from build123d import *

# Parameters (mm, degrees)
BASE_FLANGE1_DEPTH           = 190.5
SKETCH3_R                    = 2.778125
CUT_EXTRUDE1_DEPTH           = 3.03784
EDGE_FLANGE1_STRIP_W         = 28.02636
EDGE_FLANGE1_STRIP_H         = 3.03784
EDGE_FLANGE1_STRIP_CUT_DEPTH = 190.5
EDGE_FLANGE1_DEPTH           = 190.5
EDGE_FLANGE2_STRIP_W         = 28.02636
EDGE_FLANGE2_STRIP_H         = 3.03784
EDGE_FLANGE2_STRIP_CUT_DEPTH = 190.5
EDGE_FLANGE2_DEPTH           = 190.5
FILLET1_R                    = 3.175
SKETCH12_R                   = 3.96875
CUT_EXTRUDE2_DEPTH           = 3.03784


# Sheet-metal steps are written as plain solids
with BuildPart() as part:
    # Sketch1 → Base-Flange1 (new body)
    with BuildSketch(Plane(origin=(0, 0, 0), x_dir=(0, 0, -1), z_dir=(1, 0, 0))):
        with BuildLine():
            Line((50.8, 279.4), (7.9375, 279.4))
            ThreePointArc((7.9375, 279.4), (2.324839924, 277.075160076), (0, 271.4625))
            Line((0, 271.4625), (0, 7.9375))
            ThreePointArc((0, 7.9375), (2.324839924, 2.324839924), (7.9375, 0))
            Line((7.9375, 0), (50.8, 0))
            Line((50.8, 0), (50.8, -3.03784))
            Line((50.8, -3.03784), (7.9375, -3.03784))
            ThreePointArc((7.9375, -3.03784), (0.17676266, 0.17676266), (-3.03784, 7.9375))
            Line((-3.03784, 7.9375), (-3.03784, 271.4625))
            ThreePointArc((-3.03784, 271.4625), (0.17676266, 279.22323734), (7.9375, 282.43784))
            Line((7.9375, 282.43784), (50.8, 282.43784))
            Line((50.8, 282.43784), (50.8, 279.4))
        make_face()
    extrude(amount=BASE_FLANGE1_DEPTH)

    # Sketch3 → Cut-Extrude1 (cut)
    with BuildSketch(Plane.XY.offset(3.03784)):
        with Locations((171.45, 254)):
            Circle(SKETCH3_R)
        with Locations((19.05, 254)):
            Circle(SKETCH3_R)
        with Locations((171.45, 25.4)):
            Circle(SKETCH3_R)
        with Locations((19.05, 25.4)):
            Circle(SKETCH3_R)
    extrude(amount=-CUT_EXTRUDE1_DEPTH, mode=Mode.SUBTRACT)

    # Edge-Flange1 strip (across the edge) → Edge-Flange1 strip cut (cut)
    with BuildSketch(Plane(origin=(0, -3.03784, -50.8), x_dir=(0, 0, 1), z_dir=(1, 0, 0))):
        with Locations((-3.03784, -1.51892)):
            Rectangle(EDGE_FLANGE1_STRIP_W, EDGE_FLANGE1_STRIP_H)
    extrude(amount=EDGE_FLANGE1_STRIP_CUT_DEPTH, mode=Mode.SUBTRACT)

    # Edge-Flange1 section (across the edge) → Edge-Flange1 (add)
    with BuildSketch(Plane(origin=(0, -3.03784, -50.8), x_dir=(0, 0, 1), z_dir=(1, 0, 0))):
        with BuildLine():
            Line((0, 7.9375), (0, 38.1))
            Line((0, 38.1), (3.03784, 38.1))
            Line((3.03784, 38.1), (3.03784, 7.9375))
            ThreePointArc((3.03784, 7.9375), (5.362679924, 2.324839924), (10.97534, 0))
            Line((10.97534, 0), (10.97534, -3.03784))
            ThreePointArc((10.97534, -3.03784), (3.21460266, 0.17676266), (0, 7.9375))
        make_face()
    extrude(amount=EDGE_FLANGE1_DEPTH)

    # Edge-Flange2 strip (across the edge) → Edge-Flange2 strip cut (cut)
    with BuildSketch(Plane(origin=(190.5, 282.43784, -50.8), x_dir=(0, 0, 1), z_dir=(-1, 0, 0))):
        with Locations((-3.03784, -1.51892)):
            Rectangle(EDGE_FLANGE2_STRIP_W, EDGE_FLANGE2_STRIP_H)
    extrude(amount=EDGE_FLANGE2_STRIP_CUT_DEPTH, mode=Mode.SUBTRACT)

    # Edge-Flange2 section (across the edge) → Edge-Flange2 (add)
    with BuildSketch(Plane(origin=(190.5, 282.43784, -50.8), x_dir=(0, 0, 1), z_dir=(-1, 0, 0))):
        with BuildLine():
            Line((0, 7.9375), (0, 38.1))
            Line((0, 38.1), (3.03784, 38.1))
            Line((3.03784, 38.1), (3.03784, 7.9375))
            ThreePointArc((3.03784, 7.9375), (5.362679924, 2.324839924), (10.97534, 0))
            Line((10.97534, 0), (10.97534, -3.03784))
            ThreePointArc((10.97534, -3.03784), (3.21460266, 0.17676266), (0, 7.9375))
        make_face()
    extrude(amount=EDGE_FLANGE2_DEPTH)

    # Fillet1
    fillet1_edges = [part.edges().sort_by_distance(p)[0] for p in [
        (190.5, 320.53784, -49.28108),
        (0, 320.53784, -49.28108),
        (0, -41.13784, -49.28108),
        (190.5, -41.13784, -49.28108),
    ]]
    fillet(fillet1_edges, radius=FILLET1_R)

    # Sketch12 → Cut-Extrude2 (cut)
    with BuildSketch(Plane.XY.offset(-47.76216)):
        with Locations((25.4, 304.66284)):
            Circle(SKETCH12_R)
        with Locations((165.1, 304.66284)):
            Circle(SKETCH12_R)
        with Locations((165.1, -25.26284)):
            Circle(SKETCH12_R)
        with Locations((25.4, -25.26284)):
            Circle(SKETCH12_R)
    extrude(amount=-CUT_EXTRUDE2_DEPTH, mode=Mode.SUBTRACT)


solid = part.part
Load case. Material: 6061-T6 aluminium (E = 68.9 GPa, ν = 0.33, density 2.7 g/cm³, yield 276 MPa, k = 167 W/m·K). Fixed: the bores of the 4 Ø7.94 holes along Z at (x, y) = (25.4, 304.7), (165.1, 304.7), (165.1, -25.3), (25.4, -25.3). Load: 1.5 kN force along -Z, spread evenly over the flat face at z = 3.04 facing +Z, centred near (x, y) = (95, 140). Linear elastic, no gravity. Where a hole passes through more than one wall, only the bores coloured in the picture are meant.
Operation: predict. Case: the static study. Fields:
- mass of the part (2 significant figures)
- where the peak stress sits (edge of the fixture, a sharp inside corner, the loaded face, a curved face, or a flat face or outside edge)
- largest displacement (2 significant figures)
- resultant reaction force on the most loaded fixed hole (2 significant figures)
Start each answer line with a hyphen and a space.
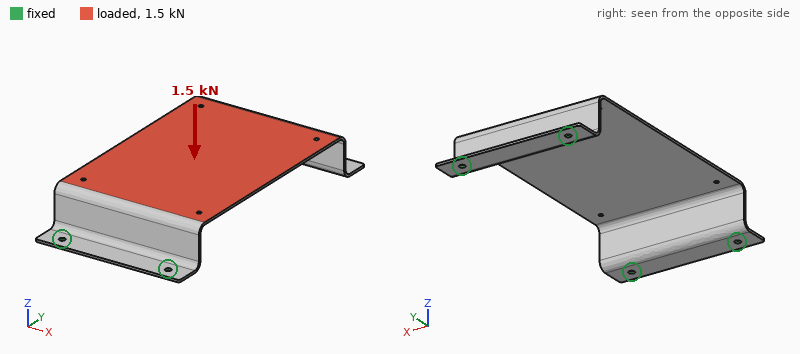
- 700 g
- a curved face
- 3.8 mm
- 640 N
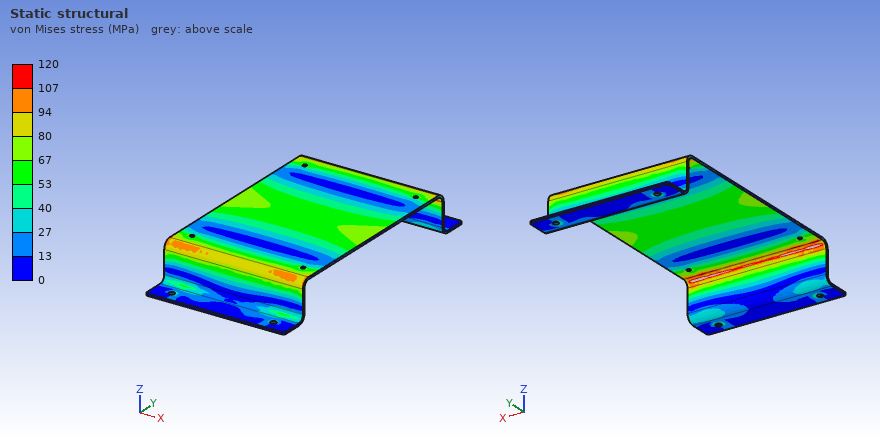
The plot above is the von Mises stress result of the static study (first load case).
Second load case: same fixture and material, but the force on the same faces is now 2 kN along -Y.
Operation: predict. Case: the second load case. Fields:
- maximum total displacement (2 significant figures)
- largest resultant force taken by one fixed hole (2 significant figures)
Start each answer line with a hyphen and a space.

- 2.0 mm
- 540 N
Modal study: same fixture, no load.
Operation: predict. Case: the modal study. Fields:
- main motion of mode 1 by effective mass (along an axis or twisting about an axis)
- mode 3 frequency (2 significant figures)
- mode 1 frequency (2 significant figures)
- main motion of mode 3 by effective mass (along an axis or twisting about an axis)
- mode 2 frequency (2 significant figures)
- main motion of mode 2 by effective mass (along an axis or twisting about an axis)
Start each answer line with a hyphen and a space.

- along Z
- 260 Hz
- 180 Hz
- twisting about Y
- 220 Hz
- along Y
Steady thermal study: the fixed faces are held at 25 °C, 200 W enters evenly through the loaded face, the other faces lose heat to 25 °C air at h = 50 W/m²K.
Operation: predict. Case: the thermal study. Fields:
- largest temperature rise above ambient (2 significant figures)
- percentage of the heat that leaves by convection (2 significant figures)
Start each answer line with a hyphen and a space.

- 53 K
- 82 %
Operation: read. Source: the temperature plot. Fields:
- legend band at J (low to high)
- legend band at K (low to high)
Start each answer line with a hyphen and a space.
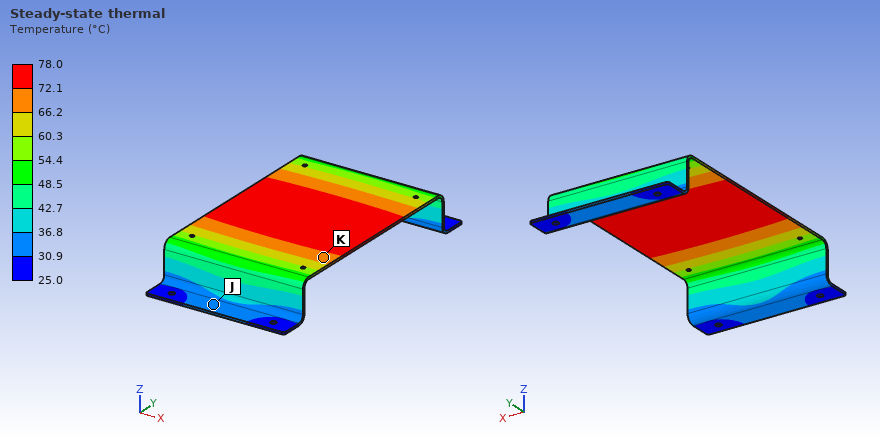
- 30.9 to 36.8 °C
- 66.2 to 72.1 °C
